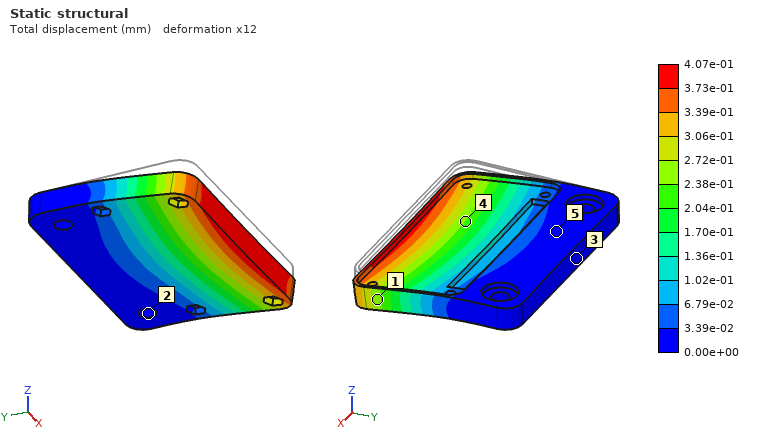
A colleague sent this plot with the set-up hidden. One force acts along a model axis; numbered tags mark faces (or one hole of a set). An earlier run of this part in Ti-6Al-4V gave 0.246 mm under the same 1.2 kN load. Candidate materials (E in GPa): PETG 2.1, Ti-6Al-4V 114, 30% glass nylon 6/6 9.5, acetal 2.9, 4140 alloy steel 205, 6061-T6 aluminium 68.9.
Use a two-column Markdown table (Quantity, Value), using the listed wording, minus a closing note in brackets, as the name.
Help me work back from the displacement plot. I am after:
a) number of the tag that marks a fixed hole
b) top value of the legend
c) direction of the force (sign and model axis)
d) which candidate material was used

| Quantity | Value |
|---|---|
| number of the tag that marks a fixed hole | 2 |
| top value of the legend | 4.07e-01 mm |
| direction of the force | -Z |
| which candidate material was used | 6061-T6 aluminium |
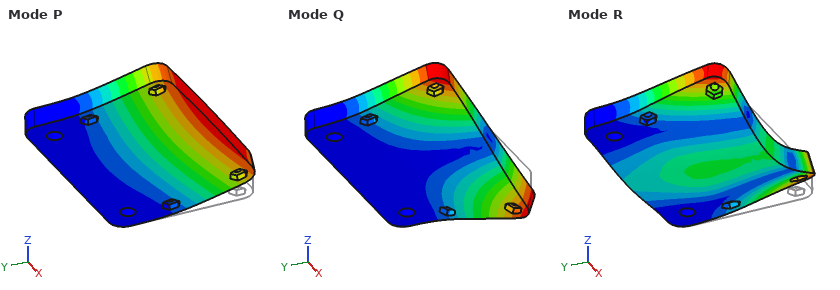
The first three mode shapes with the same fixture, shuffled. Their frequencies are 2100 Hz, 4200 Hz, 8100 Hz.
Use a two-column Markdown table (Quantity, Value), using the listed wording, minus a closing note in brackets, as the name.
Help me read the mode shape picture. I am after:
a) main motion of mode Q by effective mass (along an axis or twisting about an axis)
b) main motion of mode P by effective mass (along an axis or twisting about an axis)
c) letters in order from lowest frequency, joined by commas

| Quantity | Value |
|---|---|
| main motion of mode Q by effective mass | twisting about Y |
| main motion of mode P by effective mass | along Z |
| letters in order from lowest frequency, joined by commas | P, Q, R |
